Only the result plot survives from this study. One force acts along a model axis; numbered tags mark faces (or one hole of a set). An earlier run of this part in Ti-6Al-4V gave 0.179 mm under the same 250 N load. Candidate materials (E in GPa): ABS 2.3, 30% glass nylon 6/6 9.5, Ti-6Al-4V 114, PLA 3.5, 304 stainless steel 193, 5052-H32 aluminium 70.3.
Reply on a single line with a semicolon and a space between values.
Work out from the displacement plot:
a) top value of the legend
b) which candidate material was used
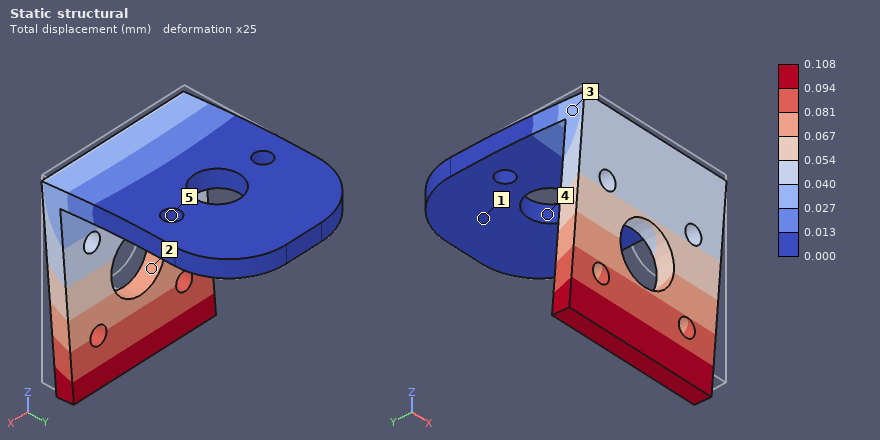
0.108 mm; 304 stainless steel
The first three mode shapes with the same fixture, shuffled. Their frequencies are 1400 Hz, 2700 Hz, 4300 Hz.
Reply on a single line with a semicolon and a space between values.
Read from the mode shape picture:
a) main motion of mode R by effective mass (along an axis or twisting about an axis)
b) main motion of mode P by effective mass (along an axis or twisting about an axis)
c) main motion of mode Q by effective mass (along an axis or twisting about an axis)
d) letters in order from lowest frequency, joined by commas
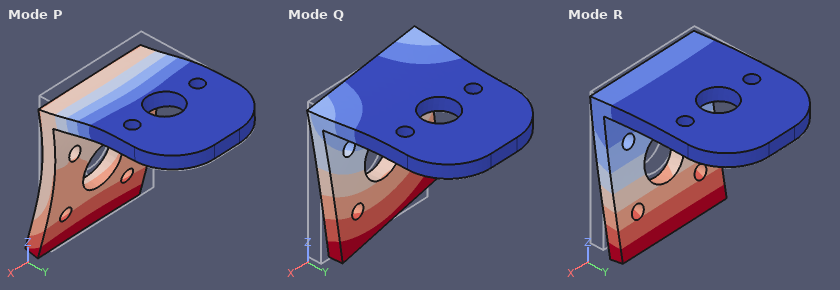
along Y; along Z; along X; R, Q, P
